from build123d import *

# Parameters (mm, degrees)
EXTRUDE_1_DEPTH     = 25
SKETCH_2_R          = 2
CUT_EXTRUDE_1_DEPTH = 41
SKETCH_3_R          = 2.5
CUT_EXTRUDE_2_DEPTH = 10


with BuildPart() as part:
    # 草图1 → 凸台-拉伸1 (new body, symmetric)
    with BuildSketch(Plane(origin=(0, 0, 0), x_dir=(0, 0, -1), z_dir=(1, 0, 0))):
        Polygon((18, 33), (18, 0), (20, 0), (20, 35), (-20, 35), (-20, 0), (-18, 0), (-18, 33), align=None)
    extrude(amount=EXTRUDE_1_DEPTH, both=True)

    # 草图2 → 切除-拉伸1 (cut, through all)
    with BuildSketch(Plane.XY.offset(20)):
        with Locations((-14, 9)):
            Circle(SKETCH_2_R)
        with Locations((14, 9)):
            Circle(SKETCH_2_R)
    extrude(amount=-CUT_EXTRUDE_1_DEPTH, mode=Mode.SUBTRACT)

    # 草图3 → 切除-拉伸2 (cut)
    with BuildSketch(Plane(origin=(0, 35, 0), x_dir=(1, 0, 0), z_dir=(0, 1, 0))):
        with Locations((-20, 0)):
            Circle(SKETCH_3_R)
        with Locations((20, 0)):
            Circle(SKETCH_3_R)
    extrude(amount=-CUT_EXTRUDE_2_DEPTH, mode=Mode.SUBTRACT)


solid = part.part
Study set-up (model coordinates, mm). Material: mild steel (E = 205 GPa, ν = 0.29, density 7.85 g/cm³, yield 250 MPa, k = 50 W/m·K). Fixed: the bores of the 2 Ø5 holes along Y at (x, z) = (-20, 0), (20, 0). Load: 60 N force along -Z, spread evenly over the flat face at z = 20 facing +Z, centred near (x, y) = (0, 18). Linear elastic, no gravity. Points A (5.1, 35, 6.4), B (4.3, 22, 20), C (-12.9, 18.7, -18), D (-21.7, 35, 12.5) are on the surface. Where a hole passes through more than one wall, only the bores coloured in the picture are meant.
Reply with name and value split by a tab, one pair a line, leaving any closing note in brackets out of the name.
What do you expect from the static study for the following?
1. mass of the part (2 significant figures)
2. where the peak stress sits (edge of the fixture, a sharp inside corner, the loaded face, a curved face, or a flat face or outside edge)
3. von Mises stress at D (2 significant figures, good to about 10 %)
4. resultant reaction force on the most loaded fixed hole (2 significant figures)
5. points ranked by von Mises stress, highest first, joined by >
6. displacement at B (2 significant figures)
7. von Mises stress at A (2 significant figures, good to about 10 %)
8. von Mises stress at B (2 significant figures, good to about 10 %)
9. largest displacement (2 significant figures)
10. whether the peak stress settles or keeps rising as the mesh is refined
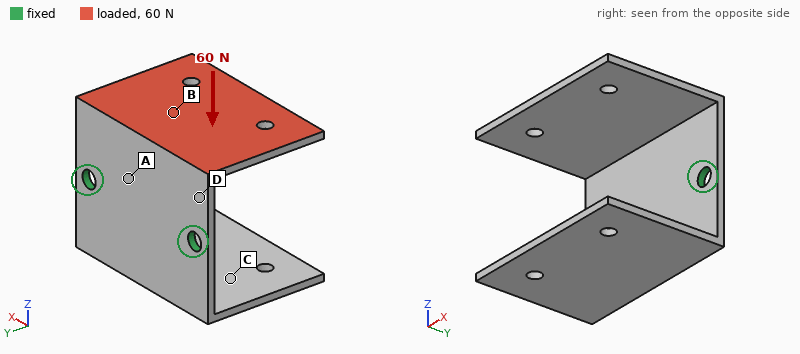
mass of the part	82 g
where the peak stress sits	edge of the fixture
von Mises stress at D	29 MPa
resultant reaction force on the most loaded fixed hole	30 N
points ranked by von Mises stress, highest first, joined by >	D > A > B > C
displacement at B	0.047 mm
von Mises stress at A	20 MPa
von Mises stress at B	11 MPa
largest displacement	0.13 mm
whether the peak stress settles or keeps rising as the mesh is refined	keeps rising
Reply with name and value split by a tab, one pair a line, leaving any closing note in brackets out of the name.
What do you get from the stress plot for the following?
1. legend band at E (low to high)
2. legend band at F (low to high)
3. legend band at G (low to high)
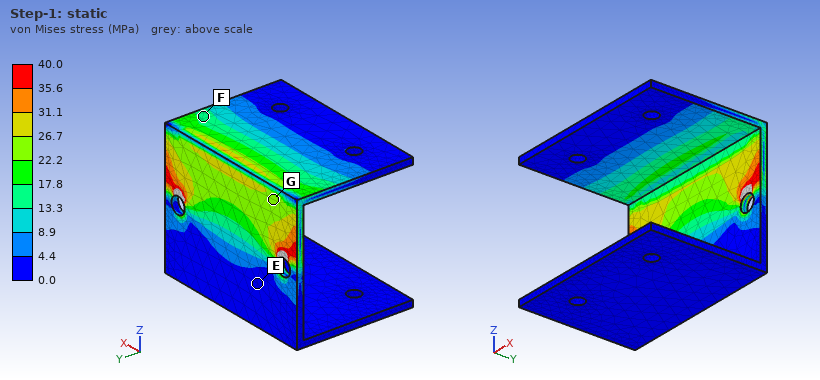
legend band at E	0.0 to 4.4 MPa
legend band at F	13.3 to 17.8 MPa
legend band at G	22.2 to 26.7 MPa
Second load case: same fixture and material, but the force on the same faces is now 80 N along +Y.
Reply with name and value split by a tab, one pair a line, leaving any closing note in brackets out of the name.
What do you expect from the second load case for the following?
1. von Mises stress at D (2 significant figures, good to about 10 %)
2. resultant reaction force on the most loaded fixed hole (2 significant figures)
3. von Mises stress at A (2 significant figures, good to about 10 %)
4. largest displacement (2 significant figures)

von Mises stress at D	20 MPa
resultant reaction force on the most loaded fixed hole	40 N
von Mises stress at A	20 MPa
largest displacement	87 µm
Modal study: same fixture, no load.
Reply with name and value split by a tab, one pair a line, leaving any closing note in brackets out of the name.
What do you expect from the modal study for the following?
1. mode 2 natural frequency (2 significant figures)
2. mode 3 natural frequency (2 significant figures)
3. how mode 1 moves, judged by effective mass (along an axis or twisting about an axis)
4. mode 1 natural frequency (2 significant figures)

mode 2 natural frequency	800 Hz
mode 3 natural frequency	1700 Hz
how mode 1 moves, judged by effective mass	along Z
mode 1 natural frequency	750 Hz
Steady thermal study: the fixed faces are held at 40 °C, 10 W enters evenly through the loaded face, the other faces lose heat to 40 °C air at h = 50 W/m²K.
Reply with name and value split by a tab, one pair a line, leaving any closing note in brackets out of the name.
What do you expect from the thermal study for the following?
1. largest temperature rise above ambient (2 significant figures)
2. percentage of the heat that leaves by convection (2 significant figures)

largest temperature rise above ambient	43 K
percentage of the heat that leaves by convection	54 %
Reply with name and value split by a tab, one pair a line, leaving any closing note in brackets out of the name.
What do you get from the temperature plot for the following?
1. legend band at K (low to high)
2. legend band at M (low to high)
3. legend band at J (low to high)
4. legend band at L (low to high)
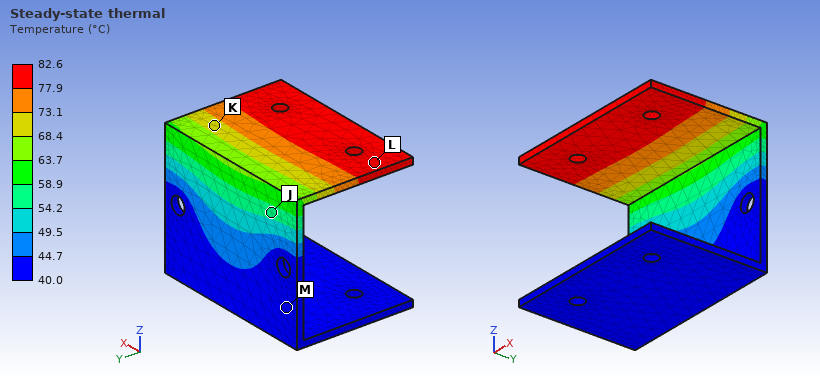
legend band at K	68.4 to 73.1 °C
legend band at M	40.0 to 44.7 °C
legend band at J	54.2 to 58.9 °C
legend band at L	77.9 to 82.6 °C
